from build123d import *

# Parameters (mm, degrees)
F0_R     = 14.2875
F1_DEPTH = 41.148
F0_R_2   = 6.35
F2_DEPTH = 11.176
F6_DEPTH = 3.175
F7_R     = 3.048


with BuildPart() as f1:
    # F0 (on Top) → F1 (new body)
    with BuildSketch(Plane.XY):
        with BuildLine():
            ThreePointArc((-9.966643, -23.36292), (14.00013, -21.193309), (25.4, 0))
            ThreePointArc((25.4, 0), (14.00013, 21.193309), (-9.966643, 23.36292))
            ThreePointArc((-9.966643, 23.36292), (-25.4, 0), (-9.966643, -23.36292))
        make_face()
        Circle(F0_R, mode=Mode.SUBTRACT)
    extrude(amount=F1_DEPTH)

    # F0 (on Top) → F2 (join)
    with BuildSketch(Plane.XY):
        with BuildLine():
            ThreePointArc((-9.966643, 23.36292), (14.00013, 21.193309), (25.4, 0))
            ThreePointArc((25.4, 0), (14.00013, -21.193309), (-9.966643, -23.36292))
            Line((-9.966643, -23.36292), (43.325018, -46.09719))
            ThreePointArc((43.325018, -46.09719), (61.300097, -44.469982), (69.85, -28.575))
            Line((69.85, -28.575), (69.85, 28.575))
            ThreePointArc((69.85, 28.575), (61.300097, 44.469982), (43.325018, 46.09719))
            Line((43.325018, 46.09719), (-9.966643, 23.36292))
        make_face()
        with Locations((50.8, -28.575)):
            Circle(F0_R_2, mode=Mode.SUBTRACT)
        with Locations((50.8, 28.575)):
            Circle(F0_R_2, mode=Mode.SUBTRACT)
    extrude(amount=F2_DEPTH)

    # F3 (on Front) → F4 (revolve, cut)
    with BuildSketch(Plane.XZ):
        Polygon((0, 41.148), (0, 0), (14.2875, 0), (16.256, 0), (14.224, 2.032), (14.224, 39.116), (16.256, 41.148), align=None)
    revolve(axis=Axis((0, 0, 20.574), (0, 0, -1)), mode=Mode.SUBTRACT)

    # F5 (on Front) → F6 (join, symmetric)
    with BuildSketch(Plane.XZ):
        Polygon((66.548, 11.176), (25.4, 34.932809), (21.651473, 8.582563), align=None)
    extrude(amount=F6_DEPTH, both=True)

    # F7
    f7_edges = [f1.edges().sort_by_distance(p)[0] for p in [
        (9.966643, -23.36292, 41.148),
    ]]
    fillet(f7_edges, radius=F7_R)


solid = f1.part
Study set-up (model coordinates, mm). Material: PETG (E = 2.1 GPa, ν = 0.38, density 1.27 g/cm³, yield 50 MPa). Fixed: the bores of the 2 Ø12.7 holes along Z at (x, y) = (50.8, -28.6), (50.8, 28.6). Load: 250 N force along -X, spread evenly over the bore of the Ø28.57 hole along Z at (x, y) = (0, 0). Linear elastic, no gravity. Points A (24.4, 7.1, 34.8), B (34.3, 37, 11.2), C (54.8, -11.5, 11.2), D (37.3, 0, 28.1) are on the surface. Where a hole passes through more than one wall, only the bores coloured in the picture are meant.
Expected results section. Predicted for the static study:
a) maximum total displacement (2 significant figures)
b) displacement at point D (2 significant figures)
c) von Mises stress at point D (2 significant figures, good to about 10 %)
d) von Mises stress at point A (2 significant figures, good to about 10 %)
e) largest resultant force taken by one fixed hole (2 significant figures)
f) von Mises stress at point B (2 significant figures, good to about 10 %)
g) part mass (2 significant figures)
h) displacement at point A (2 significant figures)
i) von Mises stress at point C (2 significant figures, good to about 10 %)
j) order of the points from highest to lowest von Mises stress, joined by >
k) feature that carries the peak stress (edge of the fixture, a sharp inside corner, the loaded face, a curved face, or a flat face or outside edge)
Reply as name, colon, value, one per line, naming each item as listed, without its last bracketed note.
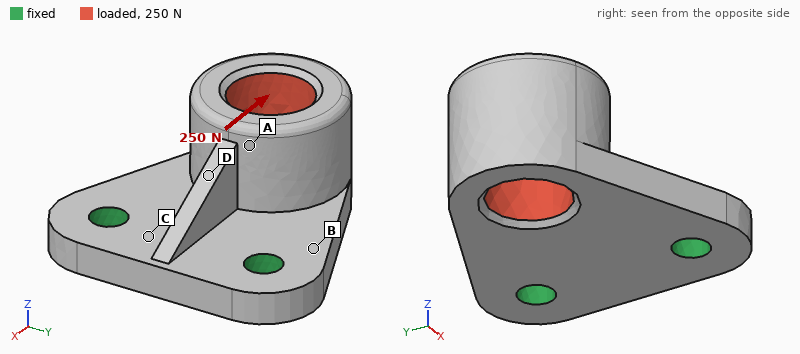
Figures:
maximum total displacement: 0.24 mm
displacement at point D: 0.067 mm
von Mises stress at point D: 1.8 MPa
von Mises stress at point A: 0.53 MPa
largest resultant force taken by one fixed hole: 130 N
von Mises stress at point B: 1.4 MPa
part mass: 140 g
displacement at point A: 0.11 mm
von Mises stress at point C: 0.84 MPa
order of the points from highest to lowest von Mises stress, joined by >: D > B > C > A
feature that carries the peak stress: a flat face or outside edge
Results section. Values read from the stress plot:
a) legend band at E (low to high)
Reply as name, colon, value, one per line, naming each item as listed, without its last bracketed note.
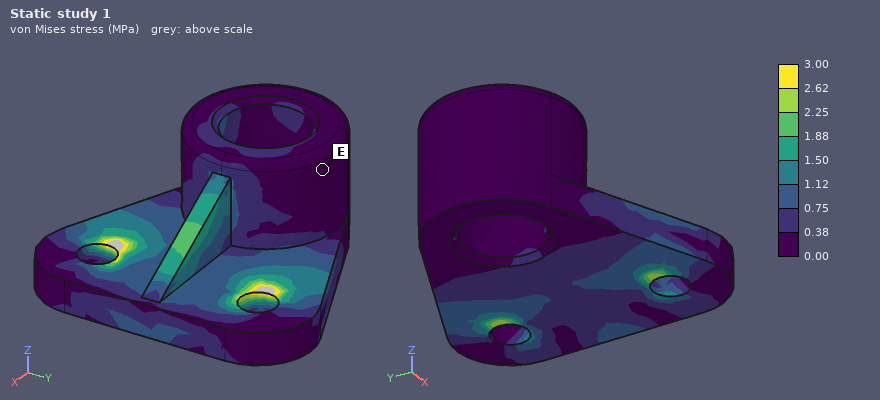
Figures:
legend band at E: 0.00 to 0.38 MPa
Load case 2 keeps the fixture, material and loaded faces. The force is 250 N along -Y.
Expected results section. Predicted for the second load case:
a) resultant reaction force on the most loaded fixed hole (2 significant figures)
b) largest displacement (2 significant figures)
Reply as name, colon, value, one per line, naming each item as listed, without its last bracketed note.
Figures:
resultant reaction force on the most loaded fixed hole: 240 N
largest displacement: 0.10 mm
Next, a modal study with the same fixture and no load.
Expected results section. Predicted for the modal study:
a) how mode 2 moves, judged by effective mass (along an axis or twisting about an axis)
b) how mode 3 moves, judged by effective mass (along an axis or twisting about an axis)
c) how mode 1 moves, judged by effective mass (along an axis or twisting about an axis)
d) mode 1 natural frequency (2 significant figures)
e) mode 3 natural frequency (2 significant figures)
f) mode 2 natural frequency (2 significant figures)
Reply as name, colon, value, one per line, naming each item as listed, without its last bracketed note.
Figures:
how mode 2 moves, judged by effective mass: along Y
how mode 3 moves, judged by effective mass: along Y
how mode 1 moves, judged by effective mass: along Z
mode 1 natural frequency: 420 Hz
mode 3 natural frequency: 1700 Hz
mode 2 natural frequency: 990 Hz
